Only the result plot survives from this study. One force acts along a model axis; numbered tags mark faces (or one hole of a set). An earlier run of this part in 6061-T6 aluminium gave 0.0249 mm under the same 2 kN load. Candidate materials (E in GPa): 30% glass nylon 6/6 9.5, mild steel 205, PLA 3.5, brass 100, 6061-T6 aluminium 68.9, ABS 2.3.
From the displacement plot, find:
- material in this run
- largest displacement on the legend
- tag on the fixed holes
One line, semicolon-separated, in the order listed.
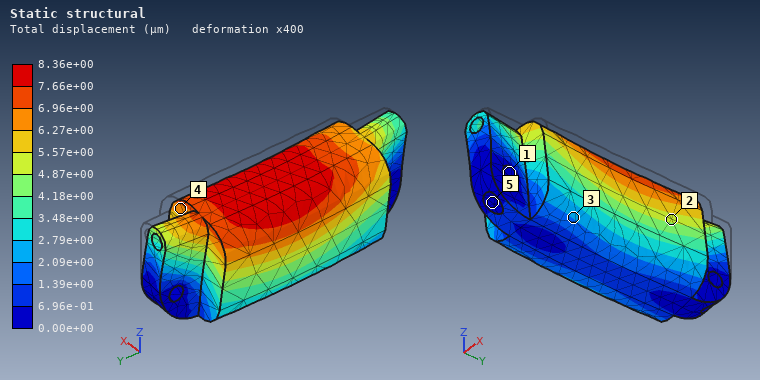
mild steel; 8.36e+00 µm; 1
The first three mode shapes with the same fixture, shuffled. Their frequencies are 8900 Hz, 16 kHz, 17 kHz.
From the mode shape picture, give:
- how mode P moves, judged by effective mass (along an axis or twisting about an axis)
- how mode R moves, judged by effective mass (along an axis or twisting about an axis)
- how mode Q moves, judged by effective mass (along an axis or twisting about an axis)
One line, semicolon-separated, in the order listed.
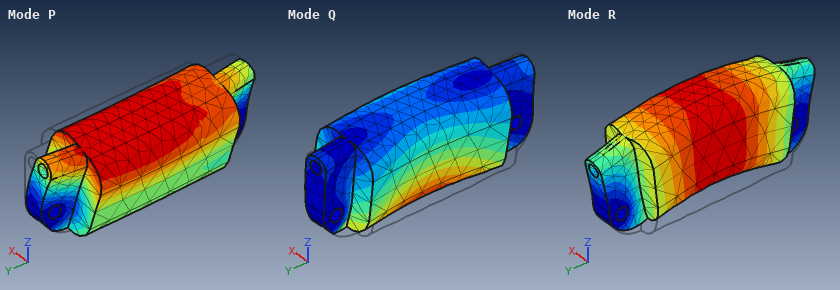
along X; along Z; along X
